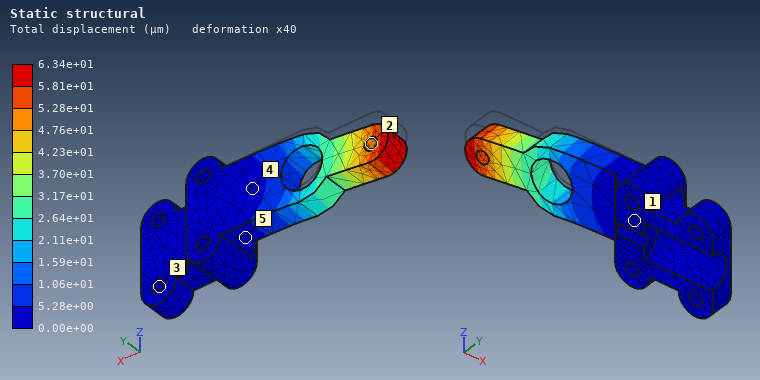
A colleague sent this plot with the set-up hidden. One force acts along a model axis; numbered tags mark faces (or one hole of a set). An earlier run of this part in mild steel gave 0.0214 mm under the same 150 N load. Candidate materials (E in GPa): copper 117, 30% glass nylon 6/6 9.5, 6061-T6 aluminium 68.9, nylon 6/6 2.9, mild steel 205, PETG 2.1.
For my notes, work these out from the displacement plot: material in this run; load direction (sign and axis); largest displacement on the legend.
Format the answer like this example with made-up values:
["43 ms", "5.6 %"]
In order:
["6061-T6 aluminium", "-Z", "6.34e+01 µm"]
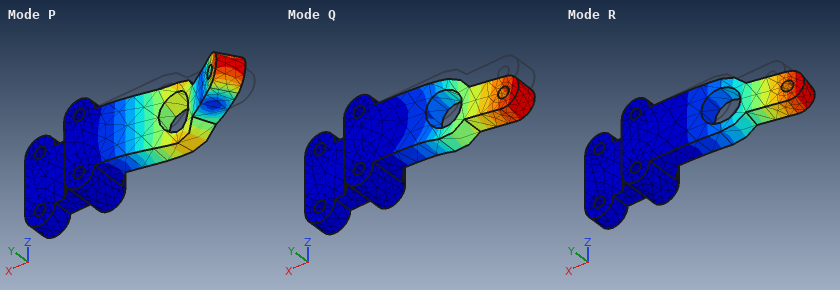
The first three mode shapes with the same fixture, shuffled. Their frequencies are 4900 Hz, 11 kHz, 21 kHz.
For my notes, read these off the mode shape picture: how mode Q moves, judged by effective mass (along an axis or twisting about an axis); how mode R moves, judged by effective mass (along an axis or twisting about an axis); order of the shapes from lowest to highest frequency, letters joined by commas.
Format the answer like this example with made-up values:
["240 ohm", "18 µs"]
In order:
["along Z", "along Y", "R, Q, P"]
